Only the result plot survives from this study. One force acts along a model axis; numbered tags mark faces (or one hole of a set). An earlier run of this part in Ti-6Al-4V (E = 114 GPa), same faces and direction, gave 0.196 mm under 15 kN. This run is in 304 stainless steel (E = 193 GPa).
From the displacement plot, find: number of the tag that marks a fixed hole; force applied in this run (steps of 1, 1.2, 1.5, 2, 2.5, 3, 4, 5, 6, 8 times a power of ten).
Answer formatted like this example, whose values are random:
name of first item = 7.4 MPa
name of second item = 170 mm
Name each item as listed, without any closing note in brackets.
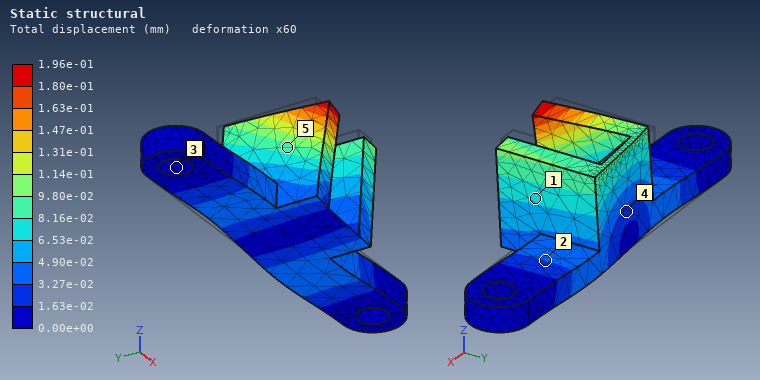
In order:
number of the tag that marks a fixed hole = 3
force applied in this run = 25 kN
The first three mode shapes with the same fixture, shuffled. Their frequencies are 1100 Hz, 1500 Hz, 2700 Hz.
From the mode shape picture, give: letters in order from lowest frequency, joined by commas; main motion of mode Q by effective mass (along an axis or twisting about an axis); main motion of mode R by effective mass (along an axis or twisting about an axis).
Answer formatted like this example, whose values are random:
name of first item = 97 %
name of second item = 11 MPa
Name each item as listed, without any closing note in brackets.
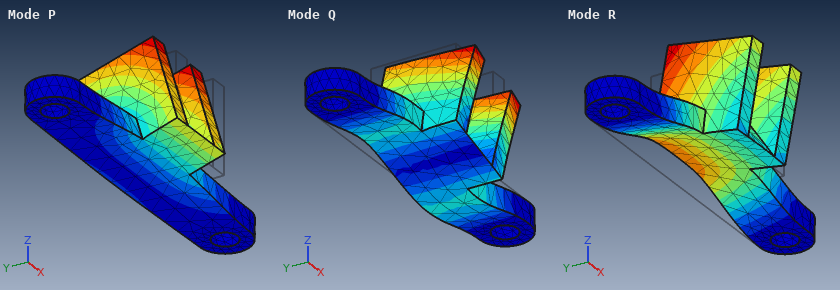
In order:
letters in order from lowest frequency, joined by commas = P, R, Q
main motion of mode Q by effective mass = along X
main motion of mode R by effective mass = along Z
